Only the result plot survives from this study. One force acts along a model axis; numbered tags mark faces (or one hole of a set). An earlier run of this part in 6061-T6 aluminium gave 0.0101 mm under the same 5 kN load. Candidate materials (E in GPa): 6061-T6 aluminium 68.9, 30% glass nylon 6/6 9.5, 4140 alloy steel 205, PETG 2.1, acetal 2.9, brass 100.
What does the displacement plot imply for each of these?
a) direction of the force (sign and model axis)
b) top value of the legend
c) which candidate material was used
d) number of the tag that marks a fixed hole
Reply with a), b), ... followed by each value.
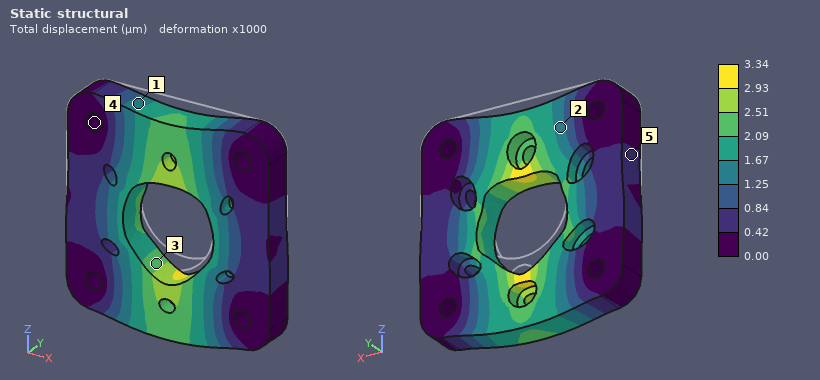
a) -Z
b) 3.34 µm
c) 4140 alloy steel
d) 4
